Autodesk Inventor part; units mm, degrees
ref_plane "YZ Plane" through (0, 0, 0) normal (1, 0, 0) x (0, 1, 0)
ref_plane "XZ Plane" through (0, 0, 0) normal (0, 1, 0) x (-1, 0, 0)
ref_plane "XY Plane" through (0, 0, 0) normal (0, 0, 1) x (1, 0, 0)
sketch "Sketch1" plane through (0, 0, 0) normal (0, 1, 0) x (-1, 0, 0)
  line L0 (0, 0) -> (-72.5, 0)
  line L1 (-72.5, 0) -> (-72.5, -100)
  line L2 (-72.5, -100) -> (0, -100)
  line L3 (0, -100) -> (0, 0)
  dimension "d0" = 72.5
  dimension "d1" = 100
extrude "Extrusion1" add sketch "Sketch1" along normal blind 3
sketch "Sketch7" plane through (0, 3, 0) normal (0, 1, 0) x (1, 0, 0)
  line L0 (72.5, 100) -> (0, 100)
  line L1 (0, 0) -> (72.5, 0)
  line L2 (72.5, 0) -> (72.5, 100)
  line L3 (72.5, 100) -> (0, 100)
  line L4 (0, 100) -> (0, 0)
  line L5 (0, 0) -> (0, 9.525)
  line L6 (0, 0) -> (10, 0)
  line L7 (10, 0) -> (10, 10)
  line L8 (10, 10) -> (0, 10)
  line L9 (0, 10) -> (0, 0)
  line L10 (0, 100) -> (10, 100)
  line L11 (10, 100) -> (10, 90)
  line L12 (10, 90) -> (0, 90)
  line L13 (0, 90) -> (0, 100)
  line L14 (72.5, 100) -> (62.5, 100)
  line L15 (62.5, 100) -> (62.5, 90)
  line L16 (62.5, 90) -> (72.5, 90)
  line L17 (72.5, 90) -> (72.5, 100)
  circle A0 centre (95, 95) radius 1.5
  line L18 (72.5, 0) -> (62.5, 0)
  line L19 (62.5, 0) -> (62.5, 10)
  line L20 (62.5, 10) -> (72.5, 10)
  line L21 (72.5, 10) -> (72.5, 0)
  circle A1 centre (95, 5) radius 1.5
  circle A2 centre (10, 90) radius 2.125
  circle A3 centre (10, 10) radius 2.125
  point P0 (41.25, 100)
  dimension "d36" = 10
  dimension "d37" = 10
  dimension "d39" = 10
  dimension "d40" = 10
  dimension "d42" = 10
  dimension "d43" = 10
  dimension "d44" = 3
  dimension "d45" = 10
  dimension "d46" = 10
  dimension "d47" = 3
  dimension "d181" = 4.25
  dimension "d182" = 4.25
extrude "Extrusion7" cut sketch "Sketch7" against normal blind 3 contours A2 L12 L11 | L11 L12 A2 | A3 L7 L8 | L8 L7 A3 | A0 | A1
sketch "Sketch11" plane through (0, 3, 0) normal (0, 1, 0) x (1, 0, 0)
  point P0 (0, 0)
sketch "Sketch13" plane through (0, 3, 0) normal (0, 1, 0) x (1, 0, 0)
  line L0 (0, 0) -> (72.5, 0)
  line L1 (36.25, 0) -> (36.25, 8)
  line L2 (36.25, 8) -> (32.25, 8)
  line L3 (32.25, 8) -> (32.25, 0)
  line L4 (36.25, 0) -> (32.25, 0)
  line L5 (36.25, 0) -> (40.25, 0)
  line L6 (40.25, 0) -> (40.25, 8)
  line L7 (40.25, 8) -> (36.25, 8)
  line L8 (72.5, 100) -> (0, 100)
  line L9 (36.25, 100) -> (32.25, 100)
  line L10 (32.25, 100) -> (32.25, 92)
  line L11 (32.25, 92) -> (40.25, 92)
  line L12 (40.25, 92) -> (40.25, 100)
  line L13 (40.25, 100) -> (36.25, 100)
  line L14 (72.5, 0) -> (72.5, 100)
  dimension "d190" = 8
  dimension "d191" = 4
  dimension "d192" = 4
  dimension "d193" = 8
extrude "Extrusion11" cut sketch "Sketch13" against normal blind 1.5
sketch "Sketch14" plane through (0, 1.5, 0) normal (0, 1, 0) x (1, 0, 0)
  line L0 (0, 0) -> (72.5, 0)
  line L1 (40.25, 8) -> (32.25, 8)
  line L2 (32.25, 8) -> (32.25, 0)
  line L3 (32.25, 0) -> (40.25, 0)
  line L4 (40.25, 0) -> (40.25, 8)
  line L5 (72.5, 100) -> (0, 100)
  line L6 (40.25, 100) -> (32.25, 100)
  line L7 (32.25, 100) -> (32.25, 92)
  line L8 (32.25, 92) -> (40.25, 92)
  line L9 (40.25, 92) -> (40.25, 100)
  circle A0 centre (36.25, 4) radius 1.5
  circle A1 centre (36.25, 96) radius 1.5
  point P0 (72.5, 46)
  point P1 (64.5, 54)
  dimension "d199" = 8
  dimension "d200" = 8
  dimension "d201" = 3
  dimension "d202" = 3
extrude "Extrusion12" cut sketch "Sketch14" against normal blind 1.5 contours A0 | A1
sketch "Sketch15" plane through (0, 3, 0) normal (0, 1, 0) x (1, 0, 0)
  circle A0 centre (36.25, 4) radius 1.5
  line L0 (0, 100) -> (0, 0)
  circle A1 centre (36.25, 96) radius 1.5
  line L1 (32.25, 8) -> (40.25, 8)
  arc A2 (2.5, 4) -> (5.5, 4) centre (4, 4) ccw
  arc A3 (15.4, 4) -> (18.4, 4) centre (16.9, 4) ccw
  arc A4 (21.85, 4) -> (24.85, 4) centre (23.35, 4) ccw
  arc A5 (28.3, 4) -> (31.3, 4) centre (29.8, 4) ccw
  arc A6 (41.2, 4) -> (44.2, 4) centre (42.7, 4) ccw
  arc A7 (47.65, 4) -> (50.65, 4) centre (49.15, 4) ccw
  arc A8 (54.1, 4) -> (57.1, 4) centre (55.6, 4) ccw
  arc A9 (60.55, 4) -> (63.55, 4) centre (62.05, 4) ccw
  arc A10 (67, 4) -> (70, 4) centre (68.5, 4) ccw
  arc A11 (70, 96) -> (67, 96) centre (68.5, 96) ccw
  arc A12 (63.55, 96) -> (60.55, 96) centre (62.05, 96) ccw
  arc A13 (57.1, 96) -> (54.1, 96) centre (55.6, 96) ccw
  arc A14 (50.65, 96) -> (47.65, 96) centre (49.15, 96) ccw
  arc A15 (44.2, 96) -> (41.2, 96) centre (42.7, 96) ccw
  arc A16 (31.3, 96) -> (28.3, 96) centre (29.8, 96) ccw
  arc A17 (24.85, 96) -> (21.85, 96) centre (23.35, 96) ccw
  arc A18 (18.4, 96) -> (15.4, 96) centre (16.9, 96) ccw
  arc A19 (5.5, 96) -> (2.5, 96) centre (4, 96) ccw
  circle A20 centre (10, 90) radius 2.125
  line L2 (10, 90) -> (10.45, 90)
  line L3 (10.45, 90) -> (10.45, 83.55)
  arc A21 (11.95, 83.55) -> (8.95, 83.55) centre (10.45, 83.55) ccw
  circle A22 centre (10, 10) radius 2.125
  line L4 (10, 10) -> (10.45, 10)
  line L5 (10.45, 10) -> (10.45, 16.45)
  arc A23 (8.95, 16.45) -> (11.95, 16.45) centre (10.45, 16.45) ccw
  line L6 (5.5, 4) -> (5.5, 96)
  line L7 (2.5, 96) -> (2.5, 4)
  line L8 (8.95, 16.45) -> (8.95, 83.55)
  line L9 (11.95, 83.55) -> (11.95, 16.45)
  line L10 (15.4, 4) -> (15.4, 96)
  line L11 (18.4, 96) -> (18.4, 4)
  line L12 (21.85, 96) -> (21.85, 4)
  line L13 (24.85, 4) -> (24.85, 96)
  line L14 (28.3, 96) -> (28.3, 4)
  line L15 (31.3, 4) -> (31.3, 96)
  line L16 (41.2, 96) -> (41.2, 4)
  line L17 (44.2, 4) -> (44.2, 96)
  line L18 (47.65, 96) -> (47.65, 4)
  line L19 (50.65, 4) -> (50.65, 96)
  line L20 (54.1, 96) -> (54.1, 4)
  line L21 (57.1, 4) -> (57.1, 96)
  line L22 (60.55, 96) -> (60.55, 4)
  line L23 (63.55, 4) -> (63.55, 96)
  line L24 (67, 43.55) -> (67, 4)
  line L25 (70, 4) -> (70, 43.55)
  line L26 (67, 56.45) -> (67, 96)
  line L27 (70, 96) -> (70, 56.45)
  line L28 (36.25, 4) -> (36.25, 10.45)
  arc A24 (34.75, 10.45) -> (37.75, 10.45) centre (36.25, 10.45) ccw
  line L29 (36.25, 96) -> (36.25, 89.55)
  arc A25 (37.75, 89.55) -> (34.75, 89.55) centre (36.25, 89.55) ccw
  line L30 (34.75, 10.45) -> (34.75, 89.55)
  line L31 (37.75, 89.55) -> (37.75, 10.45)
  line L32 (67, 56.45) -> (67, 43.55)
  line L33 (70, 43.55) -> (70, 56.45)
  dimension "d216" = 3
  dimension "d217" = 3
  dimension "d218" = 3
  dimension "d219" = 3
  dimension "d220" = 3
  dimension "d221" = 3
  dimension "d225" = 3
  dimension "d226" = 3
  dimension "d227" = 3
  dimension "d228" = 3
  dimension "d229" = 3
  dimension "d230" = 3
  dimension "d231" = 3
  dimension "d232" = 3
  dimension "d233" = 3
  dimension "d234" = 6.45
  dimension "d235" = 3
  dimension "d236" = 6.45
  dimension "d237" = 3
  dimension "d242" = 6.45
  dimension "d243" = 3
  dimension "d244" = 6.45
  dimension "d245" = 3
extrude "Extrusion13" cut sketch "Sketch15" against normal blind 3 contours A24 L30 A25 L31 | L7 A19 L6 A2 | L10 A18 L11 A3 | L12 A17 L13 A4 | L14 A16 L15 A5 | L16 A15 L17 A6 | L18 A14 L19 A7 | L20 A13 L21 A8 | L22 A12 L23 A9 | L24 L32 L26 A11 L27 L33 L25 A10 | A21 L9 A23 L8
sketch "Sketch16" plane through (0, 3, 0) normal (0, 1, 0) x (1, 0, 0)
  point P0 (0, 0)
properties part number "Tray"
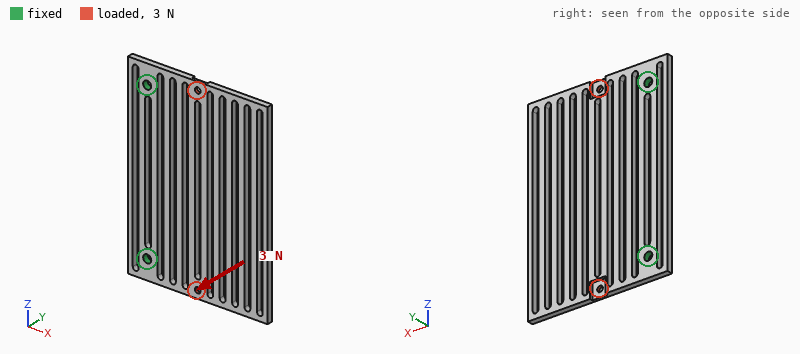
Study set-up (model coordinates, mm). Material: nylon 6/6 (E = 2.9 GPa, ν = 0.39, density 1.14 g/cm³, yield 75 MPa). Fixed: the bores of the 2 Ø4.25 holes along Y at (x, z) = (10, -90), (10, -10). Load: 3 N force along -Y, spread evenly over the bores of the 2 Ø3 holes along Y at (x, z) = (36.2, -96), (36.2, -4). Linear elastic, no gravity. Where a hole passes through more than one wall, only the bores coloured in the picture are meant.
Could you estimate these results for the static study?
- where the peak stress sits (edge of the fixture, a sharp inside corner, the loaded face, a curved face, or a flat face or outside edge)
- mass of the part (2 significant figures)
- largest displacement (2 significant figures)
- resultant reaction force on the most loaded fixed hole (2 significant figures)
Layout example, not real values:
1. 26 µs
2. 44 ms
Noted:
1. a curved face
2. 14 g
3. 1.4 mm
4. 1.5 N
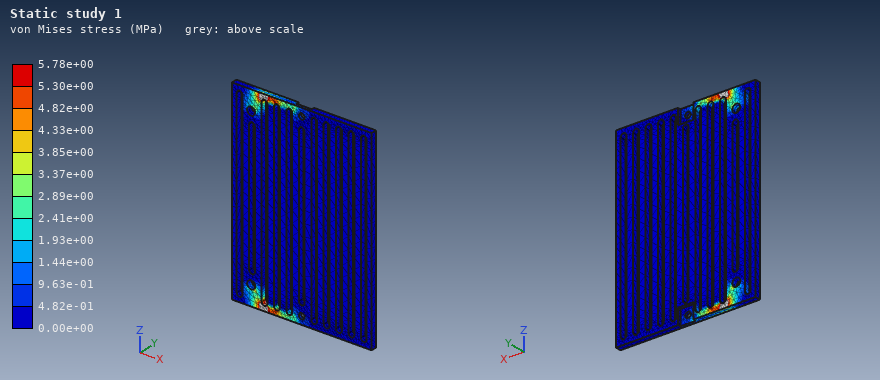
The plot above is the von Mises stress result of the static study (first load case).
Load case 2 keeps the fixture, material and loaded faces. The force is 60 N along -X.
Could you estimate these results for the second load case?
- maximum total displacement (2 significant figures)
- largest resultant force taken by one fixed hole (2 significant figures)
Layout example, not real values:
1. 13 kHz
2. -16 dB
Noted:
1. 1.2 mm
2. 30 N
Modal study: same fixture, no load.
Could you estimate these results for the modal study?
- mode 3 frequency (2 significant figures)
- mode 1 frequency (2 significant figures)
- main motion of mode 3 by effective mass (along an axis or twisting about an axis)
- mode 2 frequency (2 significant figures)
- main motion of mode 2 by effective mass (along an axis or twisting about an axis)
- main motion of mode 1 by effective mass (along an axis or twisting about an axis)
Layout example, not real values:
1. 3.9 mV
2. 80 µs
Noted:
1. 230 Hz
2. 55 Hz
3. along Y
4. 210 Hz
5. twisting about X
6. along Y
